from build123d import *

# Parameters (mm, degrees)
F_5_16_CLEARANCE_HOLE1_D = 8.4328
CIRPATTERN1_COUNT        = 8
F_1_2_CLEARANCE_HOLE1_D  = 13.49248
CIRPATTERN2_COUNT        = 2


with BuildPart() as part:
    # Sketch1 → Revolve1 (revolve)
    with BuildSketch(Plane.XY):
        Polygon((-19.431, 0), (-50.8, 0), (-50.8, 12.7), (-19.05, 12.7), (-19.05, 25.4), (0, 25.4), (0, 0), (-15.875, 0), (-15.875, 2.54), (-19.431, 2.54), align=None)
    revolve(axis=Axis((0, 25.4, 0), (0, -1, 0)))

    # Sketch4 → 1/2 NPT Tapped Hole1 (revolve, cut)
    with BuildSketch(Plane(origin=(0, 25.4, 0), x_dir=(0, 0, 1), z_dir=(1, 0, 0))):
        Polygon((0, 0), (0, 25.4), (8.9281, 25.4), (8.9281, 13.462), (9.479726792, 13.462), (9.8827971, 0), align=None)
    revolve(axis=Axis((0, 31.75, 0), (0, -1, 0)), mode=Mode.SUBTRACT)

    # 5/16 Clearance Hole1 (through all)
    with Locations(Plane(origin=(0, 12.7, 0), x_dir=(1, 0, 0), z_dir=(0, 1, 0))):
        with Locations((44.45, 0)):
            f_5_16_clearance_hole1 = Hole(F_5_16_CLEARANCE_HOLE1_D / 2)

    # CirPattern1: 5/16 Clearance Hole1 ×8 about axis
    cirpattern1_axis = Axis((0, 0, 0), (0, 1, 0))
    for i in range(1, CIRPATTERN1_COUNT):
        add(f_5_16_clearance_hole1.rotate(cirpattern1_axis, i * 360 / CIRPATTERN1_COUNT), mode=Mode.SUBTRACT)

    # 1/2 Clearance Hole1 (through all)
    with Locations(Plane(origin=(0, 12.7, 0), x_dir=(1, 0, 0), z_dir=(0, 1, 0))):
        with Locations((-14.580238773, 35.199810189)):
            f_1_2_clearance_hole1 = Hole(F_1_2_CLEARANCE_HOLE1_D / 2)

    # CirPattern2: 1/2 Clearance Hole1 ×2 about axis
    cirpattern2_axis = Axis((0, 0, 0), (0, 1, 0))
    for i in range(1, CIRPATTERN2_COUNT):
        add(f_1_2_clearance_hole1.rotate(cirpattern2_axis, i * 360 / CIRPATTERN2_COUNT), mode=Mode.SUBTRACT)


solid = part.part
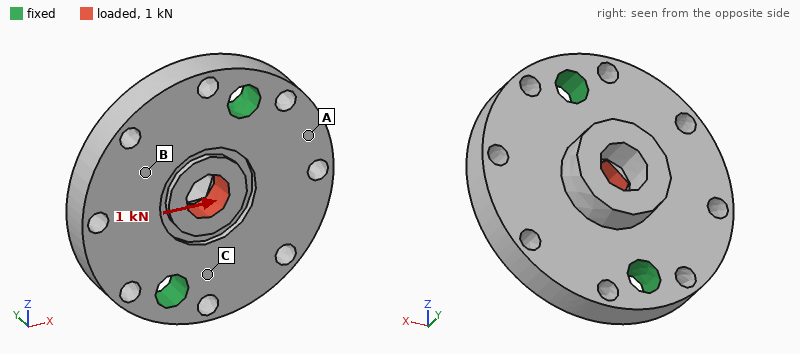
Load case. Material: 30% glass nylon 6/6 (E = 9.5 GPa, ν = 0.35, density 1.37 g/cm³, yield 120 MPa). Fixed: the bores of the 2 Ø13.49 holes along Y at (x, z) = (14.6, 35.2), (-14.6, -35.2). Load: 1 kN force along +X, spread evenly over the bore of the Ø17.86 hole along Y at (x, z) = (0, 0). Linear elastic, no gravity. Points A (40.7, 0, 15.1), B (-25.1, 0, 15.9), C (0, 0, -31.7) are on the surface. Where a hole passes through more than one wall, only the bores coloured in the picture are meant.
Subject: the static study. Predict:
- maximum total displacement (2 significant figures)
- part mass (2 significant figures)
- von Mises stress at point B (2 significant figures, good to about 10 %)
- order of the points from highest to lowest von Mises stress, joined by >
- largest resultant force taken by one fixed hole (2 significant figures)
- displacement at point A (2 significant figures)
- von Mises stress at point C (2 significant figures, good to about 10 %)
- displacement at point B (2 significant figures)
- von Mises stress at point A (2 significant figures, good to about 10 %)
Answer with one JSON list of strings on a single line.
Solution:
["8.2 µm", "140 g", "0.65 MPa", "C > B > A", "500 N", "3.5 µm", "1.2 MPa", "4.7 µm", "0.38 MPa"]
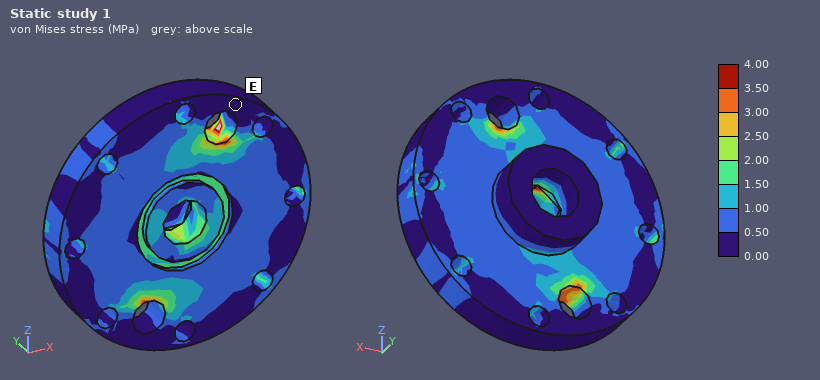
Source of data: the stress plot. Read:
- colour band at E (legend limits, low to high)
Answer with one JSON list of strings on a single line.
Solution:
["0.00 to 0.50 MPa"]
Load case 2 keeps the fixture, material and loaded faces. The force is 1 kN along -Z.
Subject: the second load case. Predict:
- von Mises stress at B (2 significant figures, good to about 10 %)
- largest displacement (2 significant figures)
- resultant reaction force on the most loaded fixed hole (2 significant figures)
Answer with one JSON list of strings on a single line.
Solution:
["0.28 MPa", "6.1 µm", "500 N"]
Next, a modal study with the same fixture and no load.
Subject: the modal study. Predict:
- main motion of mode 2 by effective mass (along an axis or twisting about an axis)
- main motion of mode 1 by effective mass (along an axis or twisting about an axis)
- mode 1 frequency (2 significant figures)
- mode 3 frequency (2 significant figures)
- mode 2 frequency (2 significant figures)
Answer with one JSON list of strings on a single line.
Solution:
["along Y", "twisting about Z", "2100 Hz", "5300 Hz", "2800 Hz"]
